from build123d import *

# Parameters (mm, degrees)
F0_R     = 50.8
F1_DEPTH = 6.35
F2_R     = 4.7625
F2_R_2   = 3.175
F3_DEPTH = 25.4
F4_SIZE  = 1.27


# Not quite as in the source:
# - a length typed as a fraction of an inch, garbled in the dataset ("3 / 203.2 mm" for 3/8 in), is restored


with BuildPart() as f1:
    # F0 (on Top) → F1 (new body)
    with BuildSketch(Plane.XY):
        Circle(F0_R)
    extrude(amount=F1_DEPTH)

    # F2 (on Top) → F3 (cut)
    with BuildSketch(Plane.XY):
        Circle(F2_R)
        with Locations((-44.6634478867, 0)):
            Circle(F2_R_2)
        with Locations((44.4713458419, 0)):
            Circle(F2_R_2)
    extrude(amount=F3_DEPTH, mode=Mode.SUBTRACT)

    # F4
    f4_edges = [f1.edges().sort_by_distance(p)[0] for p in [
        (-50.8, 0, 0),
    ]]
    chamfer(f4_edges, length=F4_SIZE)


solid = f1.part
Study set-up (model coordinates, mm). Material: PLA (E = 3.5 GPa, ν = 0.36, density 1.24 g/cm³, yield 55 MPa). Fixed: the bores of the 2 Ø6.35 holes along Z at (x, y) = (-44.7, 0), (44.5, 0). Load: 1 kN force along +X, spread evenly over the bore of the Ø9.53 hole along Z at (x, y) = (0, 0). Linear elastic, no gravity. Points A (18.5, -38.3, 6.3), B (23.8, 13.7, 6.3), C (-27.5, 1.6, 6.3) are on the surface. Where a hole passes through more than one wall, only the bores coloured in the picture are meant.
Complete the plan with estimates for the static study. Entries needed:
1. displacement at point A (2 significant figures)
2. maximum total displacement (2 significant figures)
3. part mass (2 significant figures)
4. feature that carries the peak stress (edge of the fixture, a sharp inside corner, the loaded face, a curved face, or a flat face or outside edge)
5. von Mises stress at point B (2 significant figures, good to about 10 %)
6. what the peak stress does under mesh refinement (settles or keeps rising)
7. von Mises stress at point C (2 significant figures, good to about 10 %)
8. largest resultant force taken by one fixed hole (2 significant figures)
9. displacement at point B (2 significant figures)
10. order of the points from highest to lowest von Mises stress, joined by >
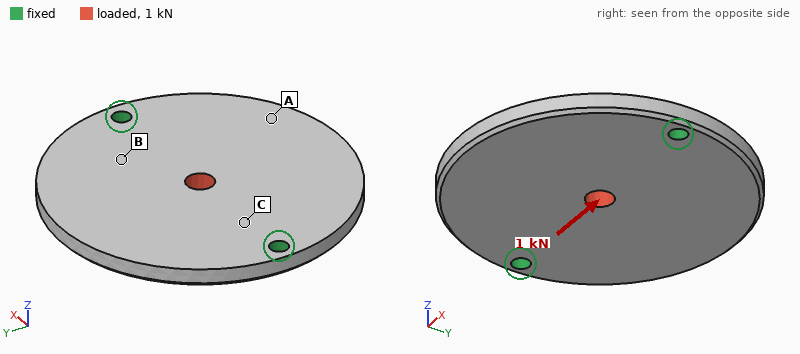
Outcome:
21 µm
44 µm
62 g
edge of the fixture
1.5 MPa
keeps rising
3.5 MPa
500 N
23 µm
C > B > A
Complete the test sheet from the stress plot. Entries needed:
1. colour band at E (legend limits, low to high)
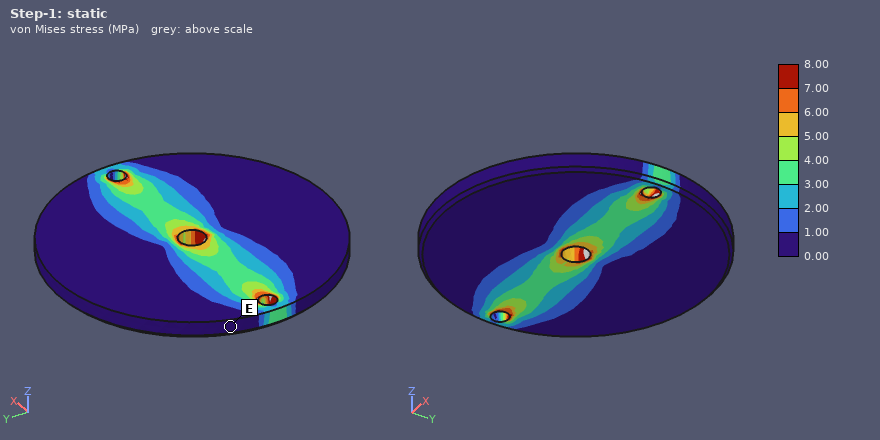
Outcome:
0.00 to 1.00 MPa
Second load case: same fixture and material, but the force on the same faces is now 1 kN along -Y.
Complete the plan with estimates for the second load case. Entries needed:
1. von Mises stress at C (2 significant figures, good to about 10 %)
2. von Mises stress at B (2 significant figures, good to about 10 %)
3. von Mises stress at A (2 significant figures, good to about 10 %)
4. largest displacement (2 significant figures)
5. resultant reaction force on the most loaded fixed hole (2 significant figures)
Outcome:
1.5 MPa
1.8 MPa
1.6 MPa
62 µm
500 N
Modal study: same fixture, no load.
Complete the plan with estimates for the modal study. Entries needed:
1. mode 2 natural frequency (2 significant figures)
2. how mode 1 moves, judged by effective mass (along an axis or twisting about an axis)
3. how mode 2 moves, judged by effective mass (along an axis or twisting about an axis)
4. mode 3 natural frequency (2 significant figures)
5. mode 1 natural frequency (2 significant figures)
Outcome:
700 Hz
twisting about X
along Z
1600 Hz
510 Hz
